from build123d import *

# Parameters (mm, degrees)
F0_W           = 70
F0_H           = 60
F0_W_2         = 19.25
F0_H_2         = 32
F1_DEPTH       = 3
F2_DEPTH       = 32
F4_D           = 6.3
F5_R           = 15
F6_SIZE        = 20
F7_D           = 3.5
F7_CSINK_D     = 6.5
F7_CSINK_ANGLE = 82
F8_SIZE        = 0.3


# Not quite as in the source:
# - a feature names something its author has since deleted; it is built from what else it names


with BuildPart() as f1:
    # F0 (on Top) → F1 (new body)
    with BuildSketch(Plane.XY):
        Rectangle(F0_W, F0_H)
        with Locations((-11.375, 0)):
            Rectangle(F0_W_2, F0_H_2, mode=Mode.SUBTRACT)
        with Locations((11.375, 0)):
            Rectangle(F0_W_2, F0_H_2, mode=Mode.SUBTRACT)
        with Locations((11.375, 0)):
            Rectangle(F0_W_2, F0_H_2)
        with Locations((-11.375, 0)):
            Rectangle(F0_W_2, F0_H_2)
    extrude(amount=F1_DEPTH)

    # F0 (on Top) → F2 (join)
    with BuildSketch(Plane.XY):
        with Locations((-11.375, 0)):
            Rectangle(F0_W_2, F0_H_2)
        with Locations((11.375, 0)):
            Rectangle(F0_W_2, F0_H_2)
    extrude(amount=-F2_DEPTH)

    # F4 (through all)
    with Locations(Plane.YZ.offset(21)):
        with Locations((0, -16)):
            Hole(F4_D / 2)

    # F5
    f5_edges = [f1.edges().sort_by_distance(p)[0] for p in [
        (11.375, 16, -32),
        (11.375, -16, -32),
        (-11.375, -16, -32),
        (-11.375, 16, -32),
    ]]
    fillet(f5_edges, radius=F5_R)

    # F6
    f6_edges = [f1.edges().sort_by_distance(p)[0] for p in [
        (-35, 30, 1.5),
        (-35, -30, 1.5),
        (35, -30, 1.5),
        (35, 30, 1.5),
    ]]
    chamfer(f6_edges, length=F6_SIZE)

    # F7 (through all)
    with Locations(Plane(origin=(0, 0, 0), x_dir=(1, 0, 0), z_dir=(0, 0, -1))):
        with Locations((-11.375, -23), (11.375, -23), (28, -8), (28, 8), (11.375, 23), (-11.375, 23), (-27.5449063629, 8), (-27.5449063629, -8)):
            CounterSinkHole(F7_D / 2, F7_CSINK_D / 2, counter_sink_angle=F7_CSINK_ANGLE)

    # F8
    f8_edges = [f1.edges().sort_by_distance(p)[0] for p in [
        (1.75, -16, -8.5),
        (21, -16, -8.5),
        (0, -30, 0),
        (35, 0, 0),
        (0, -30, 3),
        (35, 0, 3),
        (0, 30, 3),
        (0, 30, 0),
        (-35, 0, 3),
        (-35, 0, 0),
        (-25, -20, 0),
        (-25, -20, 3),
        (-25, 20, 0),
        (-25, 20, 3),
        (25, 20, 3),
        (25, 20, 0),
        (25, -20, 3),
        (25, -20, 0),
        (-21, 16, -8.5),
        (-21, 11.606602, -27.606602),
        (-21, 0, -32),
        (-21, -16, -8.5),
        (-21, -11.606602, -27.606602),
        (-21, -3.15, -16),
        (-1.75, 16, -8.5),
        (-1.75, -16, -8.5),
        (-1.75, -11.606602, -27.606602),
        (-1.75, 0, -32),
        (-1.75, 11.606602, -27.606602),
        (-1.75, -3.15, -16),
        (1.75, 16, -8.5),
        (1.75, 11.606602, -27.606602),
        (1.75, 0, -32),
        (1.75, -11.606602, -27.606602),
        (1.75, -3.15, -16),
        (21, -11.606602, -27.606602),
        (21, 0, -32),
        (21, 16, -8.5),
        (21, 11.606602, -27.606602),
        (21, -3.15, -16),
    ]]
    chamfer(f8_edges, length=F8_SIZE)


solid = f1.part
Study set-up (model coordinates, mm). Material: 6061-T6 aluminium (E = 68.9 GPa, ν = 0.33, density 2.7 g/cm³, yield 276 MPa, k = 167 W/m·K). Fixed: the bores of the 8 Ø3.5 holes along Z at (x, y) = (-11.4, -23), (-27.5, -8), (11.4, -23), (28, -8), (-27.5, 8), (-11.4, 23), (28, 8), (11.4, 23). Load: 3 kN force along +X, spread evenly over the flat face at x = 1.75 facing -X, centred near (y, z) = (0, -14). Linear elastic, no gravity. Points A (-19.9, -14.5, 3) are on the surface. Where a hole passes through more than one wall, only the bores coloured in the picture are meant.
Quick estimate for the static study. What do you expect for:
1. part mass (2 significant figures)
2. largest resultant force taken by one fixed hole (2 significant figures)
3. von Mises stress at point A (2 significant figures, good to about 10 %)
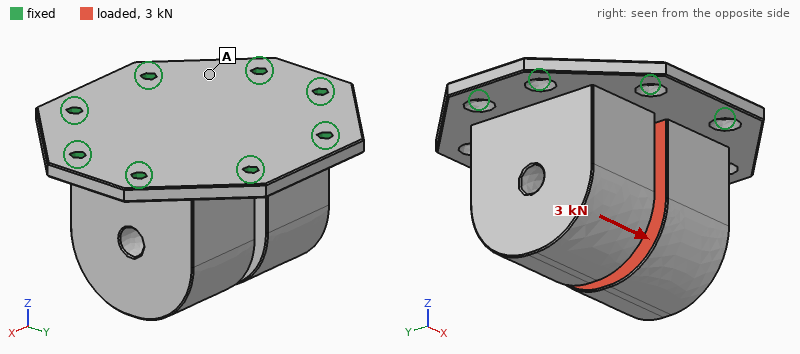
120 g
1.4 kN
23 MPa
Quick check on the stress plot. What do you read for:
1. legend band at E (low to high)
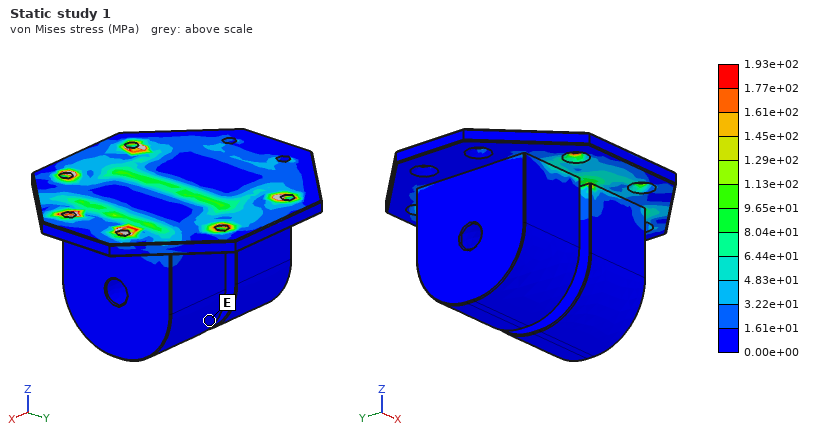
0.00e+00 to 1.61e+01 MPa
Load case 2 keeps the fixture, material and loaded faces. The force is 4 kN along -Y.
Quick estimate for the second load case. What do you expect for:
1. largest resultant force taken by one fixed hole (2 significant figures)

1.7 kN
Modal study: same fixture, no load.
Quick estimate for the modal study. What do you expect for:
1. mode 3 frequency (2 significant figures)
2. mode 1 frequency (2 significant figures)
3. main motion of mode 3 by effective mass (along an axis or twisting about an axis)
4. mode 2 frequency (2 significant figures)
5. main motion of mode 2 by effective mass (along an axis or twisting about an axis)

6200 Hz
3300 Hz
along X
5800 Hz
along Y
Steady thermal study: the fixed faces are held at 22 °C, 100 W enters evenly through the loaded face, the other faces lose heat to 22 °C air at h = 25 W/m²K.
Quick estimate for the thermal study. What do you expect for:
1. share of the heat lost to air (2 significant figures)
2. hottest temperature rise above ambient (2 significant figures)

4.7 %
43 K
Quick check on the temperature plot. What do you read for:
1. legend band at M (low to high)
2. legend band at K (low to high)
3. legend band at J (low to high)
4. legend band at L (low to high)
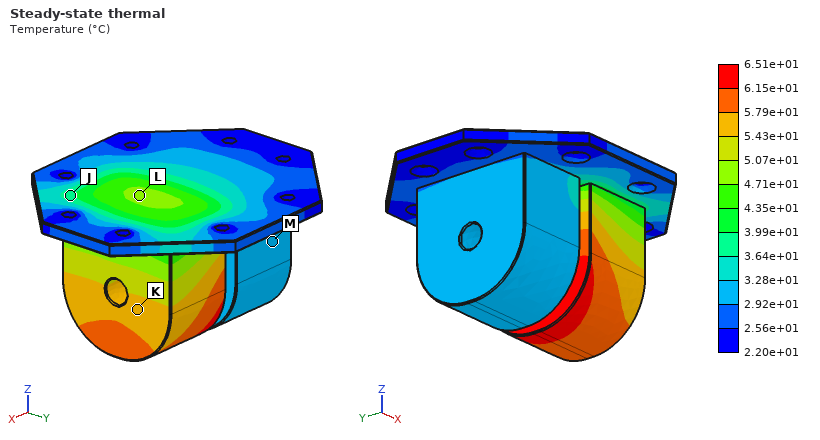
2.92e+01 to 3.28e+01 °C
5.43e+01 to 5.79e+01 °C
3.64e+01 to 3.99e+01 °C
4.71e+01 to 5.07e+01 °C
